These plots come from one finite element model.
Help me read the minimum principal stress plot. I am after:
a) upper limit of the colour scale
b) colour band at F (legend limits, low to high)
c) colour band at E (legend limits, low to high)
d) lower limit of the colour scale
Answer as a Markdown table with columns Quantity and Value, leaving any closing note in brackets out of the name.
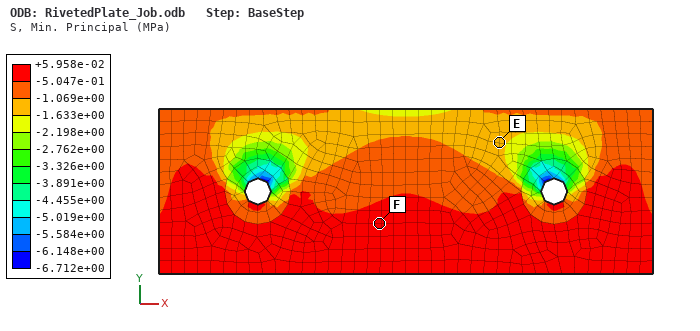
| Quantity | Value |
|---|---|
| upper limit of the colour scale | +5.958e-02 MPa |
| colour band at F | -5.047e-01 to +5.958e-02 MPa |
| colour band at E | -1.633e+00 to -1.069e+00 MPa |
| lower limit of the colour scale | -6.712e+00 MPa |
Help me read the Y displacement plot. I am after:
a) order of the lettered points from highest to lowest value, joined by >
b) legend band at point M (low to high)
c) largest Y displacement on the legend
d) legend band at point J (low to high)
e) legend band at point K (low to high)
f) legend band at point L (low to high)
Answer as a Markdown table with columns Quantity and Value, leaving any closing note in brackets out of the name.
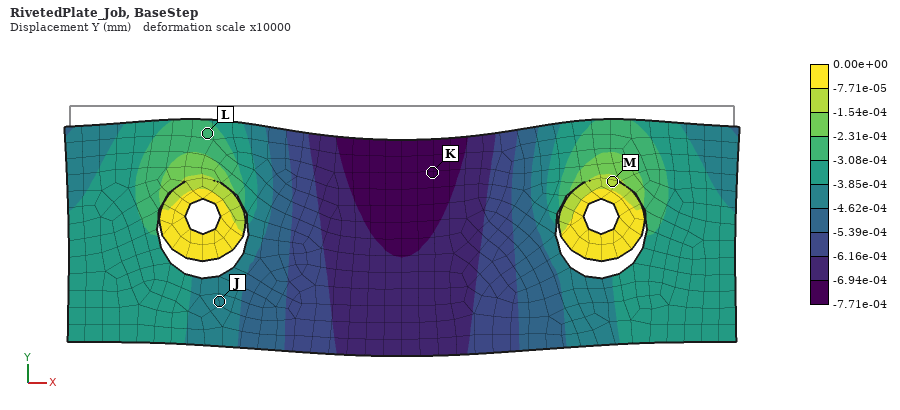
| Quantity | Value |
|---|---|
| order of the lettered points from highest to lowest value, joined by > | M > L > J > K |
| legend band at point M | -1.54e-04 to -7.71e-05 mm |
| largest Y displacement on the legend | 0.00e+00 mm |
| legend band at point J | -4.62e-04 to -3.85e-04 mm |
| legend band at point K | -7.71e-04 to -6.94e-04 mm |
| legend band at point L | -3.08e-04 to -2.31e-04 mm |
